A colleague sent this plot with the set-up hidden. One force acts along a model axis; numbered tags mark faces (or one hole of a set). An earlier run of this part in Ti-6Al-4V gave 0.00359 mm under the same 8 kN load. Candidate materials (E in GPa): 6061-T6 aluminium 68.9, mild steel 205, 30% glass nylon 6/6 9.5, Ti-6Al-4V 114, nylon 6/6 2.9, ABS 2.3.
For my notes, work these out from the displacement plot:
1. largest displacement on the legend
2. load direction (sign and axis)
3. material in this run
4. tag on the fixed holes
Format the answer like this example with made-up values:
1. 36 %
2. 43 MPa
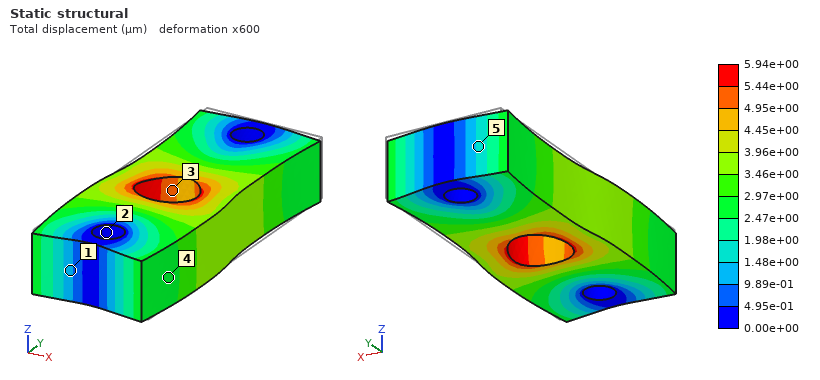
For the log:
1. 5.94e+00 µm
2. -Y
3. 6061-T6 aluminium
4. 2
